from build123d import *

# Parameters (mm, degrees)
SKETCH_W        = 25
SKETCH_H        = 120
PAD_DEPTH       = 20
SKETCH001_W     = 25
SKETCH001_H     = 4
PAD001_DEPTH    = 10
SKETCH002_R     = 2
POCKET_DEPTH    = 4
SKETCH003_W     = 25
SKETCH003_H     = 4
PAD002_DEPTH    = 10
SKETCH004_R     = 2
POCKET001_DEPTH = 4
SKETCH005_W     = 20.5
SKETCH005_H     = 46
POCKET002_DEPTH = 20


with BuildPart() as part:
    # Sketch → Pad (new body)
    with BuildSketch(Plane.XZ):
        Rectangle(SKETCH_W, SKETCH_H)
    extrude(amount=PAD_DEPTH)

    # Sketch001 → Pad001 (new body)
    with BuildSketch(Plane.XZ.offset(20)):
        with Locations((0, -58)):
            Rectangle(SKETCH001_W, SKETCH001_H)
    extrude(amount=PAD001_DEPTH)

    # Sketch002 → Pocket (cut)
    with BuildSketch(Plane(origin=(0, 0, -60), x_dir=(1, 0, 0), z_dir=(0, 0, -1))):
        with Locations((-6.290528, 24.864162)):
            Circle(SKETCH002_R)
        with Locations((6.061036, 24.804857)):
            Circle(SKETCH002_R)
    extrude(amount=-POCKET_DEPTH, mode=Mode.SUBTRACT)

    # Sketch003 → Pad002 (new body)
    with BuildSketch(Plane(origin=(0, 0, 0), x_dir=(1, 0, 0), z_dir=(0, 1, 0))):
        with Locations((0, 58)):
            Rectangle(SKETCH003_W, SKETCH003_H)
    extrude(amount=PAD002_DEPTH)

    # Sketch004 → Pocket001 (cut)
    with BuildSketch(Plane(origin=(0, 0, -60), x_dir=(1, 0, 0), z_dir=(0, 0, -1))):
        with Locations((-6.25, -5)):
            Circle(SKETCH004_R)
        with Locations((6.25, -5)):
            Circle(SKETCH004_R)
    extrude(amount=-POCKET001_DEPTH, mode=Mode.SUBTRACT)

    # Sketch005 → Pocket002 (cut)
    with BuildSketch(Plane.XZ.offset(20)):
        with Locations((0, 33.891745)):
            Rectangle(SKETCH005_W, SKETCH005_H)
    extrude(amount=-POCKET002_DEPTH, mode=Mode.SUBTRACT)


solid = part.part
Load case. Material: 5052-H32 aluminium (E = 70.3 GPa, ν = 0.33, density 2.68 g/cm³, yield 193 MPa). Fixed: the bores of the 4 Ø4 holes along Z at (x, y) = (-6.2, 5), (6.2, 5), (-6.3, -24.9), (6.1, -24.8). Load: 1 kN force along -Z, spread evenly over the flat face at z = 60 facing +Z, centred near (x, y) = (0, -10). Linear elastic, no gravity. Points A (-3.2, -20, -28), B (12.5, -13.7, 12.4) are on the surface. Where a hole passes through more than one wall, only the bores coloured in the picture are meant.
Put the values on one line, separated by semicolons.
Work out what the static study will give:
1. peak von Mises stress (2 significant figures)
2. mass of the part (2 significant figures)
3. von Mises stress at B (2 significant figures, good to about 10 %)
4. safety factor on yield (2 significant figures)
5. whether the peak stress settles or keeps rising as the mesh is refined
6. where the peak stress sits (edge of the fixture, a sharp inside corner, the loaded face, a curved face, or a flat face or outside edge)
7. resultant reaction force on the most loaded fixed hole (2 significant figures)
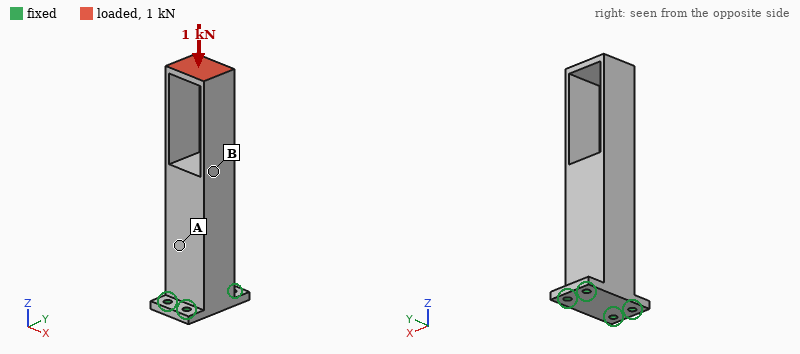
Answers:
66 MPa; 120 g; 20 MPa; 2.9; settles; a flat face or outside edge; 280 N
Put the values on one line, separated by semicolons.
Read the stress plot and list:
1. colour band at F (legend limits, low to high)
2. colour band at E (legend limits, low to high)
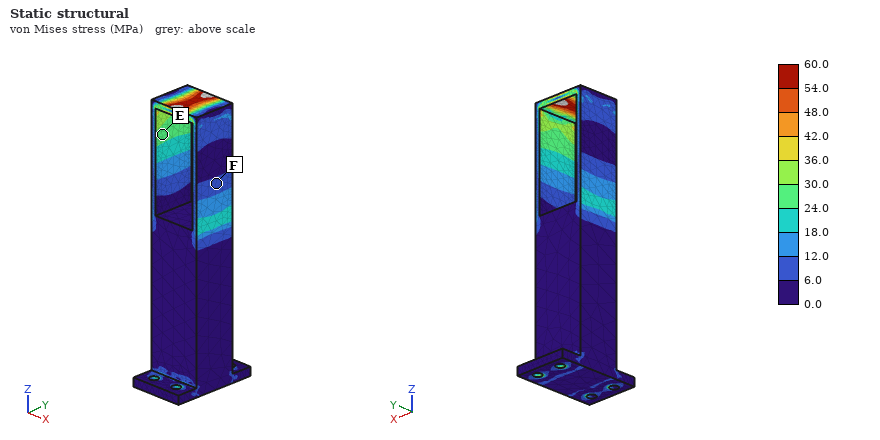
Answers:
6.0 to 12.0 MPa; 24.0 to 30.0 MPa
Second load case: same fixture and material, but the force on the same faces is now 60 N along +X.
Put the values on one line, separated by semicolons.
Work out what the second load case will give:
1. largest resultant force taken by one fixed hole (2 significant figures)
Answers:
240 N
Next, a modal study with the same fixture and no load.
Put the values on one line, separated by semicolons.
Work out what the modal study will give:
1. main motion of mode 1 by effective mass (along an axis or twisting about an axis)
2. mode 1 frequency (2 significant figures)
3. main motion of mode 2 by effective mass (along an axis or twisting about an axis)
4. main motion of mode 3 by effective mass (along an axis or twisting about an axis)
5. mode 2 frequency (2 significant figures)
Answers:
along X; 790 Hz; along Y; along X; 1500 Hz
